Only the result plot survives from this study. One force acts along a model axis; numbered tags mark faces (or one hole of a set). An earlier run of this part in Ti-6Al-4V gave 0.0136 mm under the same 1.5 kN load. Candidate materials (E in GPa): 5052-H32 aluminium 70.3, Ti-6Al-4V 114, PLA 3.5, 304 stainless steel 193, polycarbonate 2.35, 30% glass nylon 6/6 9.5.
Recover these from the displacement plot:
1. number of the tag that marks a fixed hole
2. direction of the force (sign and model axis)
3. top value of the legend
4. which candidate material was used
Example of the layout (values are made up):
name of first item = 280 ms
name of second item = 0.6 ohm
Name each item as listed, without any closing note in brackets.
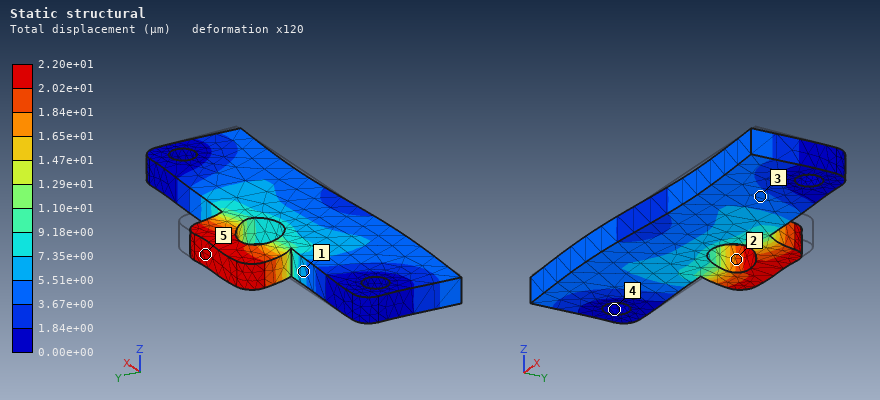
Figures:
number of the tag that marks a fixed hole = 4
direction of the force = -X
top value of the legend = 2.20e+01 µm
which candidate material was used = 5052-H32 aluminium
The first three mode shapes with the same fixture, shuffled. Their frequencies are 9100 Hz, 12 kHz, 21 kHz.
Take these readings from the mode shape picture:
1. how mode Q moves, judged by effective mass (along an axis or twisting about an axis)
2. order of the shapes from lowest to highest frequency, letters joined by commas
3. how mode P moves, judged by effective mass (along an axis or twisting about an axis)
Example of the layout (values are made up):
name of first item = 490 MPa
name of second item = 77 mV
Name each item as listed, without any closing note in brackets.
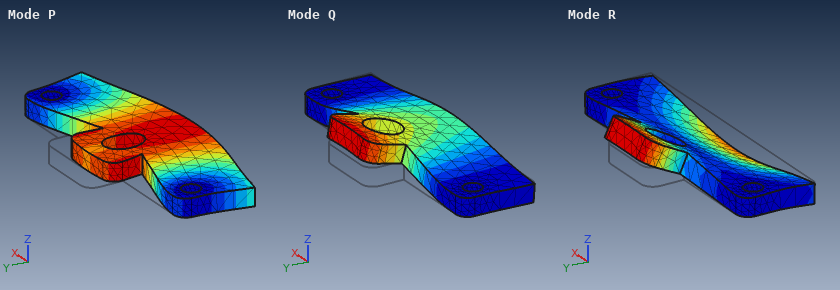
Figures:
how mode Q moves, judged by effective mass = along Z
order of the shapes from lowest to highest frequency, letters joined by commas = Q, R, P
how mode P moves, judged by effective mass = along Y
